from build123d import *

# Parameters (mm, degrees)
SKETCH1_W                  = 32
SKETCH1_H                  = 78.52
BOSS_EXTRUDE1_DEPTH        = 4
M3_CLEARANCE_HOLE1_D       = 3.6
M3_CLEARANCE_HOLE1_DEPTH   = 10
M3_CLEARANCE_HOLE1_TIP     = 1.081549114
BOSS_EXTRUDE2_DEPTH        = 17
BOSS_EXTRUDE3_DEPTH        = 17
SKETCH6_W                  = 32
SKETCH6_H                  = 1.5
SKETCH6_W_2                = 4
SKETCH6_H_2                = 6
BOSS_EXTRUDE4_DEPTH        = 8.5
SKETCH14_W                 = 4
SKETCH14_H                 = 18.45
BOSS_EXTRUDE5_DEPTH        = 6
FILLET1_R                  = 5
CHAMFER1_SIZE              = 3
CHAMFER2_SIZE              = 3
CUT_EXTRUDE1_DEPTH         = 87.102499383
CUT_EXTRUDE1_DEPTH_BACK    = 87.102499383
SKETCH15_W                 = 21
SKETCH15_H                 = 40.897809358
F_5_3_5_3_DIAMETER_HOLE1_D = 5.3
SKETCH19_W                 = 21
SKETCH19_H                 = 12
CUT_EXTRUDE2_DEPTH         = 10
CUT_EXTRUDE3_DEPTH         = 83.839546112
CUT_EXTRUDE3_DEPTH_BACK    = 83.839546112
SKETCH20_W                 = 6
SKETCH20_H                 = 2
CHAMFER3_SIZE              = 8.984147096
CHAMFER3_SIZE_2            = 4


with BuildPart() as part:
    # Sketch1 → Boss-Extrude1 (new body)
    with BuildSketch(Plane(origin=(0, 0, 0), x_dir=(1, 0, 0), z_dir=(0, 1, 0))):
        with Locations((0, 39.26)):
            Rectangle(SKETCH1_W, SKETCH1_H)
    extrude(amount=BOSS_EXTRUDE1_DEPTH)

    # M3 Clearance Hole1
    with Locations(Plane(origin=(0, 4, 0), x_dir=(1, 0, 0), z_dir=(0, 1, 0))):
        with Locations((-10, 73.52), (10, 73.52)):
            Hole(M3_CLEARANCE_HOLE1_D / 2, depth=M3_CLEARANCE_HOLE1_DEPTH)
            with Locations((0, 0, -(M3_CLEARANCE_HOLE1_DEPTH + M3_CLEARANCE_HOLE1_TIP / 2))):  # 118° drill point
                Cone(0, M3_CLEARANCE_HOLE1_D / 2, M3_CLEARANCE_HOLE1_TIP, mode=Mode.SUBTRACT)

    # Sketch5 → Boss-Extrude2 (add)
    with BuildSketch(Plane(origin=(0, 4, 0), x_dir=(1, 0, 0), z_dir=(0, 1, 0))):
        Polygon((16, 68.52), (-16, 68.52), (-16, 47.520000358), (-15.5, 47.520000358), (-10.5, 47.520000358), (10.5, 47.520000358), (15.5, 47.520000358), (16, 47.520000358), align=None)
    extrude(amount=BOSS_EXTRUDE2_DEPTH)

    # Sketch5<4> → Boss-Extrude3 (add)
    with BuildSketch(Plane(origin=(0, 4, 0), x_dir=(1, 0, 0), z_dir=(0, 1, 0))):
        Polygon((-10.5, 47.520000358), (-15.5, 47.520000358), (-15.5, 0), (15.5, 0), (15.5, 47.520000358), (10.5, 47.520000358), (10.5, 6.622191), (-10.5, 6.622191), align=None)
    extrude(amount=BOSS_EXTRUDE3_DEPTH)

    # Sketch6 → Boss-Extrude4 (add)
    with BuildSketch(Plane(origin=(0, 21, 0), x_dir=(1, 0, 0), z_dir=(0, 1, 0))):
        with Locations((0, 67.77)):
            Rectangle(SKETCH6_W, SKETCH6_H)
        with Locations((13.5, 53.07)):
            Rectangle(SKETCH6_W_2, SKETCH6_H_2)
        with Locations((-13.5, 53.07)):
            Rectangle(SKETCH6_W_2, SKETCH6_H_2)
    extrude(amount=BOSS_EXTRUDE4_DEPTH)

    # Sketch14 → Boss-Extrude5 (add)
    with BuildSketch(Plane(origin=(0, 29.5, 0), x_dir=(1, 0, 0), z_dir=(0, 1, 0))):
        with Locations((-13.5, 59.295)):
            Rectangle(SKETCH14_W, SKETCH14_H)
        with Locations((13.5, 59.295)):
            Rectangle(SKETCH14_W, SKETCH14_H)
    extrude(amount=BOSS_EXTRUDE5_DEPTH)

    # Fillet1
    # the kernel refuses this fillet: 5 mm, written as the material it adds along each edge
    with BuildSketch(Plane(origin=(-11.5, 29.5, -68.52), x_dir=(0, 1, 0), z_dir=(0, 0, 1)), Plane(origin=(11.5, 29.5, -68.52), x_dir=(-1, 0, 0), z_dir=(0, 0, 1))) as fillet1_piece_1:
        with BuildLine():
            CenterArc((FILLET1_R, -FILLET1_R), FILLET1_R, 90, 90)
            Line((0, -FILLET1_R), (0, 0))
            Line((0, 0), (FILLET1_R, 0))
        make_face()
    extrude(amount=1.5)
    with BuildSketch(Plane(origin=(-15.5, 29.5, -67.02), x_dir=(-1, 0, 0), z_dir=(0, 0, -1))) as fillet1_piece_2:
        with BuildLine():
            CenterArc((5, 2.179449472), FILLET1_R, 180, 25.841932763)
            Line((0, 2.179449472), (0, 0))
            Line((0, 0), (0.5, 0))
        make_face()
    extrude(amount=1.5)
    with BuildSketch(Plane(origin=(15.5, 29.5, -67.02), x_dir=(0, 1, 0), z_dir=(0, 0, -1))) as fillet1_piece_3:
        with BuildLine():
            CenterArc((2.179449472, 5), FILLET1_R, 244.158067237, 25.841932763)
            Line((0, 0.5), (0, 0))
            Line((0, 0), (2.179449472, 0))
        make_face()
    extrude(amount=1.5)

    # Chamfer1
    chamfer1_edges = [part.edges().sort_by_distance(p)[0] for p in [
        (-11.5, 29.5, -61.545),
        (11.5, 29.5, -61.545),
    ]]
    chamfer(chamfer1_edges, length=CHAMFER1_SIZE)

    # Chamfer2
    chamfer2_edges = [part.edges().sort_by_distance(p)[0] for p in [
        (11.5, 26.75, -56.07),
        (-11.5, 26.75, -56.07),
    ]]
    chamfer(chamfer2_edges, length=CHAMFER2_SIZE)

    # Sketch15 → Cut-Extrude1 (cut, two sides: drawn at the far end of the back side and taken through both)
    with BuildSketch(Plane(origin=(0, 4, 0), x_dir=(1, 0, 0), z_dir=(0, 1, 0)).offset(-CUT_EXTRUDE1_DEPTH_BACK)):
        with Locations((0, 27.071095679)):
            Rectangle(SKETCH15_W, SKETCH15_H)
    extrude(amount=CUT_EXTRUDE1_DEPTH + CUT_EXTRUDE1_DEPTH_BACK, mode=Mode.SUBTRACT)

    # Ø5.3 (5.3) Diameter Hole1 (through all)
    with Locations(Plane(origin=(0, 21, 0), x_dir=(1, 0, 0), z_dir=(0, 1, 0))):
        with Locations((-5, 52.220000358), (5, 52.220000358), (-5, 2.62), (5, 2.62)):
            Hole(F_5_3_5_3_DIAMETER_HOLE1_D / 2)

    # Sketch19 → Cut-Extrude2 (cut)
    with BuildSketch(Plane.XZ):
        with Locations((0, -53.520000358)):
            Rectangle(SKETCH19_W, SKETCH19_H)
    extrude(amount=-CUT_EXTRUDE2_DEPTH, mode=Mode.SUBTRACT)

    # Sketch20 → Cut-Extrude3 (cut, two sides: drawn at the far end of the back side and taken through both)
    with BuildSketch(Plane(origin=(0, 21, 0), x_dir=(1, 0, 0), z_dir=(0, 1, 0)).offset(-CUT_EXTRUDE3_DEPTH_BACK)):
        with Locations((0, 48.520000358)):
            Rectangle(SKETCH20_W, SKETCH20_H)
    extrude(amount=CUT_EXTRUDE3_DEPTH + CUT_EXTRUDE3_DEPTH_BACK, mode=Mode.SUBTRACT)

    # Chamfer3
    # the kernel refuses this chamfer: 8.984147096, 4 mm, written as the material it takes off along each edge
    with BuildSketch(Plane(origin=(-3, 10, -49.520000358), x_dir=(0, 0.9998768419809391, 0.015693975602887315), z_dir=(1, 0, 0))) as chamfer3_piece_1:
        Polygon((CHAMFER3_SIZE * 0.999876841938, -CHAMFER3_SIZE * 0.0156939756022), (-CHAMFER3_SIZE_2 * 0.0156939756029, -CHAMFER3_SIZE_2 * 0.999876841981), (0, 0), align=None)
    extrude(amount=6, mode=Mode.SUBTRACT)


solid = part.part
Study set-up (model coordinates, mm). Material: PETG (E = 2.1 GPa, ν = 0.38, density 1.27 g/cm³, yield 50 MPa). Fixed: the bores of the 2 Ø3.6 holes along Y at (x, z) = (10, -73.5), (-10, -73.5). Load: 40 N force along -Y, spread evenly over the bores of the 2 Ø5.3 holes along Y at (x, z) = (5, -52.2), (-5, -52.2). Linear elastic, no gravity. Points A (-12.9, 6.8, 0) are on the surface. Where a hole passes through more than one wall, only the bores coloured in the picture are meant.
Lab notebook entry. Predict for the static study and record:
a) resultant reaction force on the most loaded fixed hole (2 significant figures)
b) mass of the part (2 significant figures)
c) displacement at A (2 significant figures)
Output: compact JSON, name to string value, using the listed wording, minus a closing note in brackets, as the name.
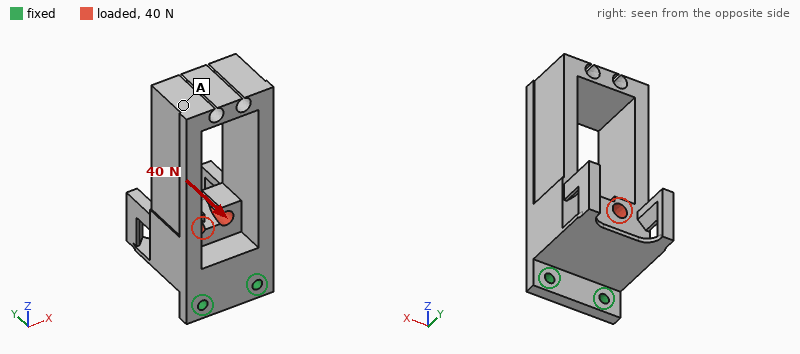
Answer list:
{"resultant reaction force on the most loaded fixed hole": "20 N", "mass of the part": "33 g", "displacement at A": "0.98 mm"}
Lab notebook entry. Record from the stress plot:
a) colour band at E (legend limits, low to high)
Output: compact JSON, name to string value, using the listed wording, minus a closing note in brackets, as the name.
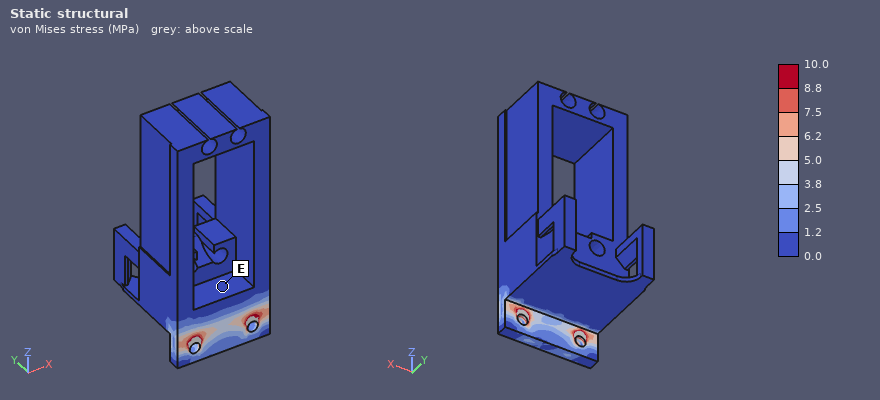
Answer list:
{"colour band at E": "0.0 to 1.2 MPa"}
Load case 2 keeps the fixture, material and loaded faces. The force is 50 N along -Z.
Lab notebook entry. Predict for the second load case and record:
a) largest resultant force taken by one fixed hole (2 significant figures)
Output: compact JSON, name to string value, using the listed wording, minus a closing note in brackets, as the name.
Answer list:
{"largest resultant force taken by one fixed hole": "26 N"}
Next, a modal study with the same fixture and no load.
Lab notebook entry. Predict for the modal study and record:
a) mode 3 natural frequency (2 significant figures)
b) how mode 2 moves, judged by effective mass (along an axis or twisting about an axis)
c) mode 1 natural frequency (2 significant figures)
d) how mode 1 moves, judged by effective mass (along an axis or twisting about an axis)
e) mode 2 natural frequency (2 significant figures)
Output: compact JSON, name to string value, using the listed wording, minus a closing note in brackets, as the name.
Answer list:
{"mode 3 natural frequency": "840 Hz", "how mode 2 moves, judged by effective mass": "along X", "mode 1 natural frequency": "160 Hz", "how mode 1 moves, judged by effective mass": "along Y", "mode 2 natural frequency": "360 Hz"}
